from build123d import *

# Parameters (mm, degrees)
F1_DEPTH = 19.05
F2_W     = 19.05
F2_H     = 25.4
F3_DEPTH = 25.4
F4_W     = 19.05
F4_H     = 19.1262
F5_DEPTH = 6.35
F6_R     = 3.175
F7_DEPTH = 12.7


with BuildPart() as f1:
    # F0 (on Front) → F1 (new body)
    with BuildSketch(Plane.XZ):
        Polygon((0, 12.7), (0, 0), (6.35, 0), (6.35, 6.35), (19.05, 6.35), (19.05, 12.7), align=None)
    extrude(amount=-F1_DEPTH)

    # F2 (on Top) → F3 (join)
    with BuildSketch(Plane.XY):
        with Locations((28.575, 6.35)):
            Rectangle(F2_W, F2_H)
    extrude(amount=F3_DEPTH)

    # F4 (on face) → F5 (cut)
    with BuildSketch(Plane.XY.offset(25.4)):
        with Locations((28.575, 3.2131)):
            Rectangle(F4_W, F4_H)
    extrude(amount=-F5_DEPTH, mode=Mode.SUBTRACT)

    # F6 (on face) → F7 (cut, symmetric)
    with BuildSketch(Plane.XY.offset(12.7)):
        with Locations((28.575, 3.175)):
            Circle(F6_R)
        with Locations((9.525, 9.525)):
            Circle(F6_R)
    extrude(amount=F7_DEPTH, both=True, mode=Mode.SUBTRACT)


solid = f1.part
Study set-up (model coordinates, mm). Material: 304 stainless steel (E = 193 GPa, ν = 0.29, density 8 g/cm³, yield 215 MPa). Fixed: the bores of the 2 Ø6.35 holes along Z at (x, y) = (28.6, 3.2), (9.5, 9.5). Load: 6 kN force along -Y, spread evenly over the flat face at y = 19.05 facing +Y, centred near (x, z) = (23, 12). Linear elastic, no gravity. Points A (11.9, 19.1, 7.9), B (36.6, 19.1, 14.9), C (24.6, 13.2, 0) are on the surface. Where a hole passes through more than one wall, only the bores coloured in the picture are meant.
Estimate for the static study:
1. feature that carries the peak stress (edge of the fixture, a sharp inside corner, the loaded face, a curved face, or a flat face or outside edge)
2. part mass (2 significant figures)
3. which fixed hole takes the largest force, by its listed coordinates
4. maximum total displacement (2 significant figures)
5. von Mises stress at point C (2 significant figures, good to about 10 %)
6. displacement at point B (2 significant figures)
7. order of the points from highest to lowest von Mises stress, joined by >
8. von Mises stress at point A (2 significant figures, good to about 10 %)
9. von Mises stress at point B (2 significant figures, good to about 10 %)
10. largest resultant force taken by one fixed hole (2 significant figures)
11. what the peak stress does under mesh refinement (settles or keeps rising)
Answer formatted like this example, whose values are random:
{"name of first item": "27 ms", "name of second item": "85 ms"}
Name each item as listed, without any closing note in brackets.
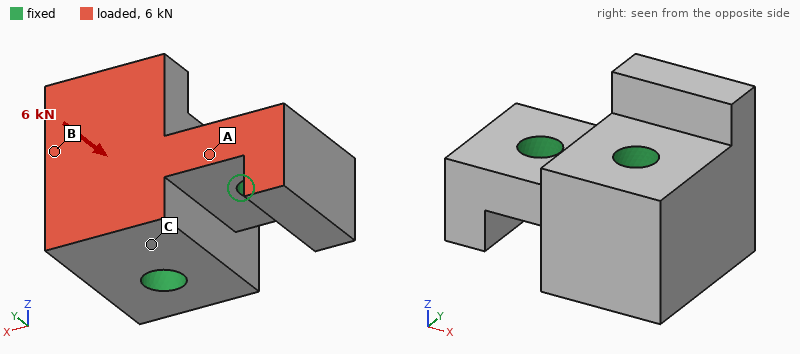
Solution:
{"feature that carries the peak stress": "edge of the fixture", "part mass": "98 g", "which fixed hole takes the largest force, by its listed coordinates": "(28.6, 3.2)", "maximum total displacement": "5.4 µm", "von Mises stress at point C": "7.4 MPa", "displacement at point B": "1.9 µm", "order of the points from highest to lowest von Mises stress, joined by >": "B > A > C", "von Mises stress at point A": "17 MPa", "von Mises stress at point B": "28 MPa", "largest resultant force taken by one fixed hole": "4.4 kN", "what the peak stress does under mesh refinement": "keeps rising"}
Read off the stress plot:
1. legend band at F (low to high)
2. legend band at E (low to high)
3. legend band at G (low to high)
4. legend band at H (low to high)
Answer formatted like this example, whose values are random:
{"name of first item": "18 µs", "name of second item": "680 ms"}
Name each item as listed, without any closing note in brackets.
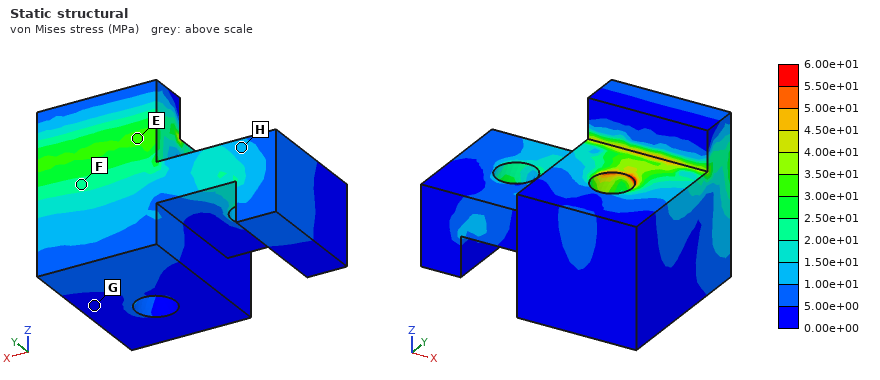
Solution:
{"legend band at F": "2.00e+01 to 2.50e+01 MPa", "legend band at E": "3.00e+01 to 3.50e+01 MPa", "legend band at G": "0.00e+00 to 5.00e+00 MPa", "legend band at H": "1.00e+01 to 1.50e+01 MPa"}
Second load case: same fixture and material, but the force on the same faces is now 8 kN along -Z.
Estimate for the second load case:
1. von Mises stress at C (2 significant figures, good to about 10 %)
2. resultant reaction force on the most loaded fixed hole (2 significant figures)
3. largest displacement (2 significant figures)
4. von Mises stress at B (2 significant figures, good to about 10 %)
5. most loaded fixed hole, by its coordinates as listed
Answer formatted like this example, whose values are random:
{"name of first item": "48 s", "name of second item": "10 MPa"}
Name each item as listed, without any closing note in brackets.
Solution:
{"von Mises stress at C": "32 MPa", "resultant reaction force on the most loaded fixed hole": "5.5 kN", "largest displacement": "14 µm", "von Mises stress at B": "48 MPa", "most loaded fixed hole, by its coordinates as listed": "(28.6, 3.2)"}
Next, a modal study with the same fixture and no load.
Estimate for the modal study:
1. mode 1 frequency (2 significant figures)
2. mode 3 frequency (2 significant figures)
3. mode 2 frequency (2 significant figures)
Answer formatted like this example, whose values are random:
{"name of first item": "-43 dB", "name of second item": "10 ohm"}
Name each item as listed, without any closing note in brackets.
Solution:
{"mode 1 frequency": "28 kHz", "mode 3 frequency": "31 kHz", "mode 2 frequency": "29 kHz"}
